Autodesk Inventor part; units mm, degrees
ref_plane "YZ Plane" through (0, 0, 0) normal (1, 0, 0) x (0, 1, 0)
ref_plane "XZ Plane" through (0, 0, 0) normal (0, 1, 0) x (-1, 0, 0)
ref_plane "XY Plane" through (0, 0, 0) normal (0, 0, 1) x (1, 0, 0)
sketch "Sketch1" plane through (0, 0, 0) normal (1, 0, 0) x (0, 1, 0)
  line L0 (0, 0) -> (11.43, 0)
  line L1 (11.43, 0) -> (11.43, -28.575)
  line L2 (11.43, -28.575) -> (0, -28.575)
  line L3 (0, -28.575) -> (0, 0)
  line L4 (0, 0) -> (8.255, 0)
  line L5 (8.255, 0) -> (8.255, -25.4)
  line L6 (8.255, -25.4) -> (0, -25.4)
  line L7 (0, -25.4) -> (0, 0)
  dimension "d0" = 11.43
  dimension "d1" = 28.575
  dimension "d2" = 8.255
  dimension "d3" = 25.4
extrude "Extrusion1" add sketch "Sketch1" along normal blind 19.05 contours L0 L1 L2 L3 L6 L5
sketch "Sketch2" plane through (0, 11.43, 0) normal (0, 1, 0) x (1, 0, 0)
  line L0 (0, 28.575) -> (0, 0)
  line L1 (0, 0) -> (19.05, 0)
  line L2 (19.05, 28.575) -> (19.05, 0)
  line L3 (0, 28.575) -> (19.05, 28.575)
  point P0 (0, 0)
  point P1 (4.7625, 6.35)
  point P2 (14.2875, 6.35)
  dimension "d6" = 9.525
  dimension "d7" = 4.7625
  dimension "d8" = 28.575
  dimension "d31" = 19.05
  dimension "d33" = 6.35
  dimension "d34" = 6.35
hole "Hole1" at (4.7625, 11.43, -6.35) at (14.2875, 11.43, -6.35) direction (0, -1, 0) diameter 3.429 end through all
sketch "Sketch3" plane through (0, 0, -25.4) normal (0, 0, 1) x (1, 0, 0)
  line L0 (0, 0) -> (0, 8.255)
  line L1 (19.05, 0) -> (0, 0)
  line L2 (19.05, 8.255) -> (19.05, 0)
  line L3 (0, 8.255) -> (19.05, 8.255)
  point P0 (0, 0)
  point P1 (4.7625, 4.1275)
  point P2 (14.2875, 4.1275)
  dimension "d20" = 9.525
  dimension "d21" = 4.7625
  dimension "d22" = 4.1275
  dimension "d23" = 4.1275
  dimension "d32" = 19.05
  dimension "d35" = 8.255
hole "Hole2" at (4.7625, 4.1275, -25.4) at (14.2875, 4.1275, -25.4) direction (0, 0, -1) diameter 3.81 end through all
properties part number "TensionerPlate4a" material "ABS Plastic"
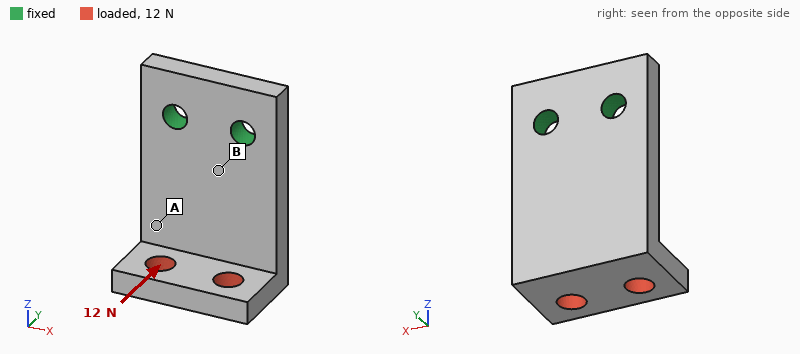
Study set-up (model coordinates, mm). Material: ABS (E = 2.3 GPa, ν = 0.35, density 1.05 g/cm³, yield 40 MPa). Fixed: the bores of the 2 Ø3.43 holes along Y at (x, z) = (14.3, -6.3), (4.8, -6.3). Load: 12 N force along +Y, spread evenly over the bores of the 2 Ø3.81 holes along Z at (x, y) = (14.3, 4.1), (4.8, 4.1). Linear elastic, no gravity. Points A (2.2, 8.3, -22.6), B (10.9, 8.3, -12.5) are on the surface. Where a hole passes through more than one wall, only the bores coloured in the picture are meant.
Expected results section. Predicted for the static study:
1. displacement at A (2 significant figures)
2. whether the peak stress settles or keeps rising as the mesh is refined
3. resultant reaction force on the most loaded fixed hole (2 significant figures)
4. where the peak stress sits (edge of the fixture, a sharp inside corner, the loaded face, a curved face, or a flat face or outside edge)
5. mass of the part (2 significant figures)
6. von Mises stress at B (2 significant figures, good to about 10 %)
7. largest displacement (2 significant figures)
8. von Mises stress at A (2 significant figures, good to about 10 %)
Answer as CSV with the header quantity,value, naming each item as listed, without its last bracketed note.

quantity,value
displacement at A,0.18 mm
whether the peak stress settles or keeps rising as the mesh is refined,keeps rising
resultant reaction force on the most loaded fixed hole,6.0 N
where the peak stress sits,edge of the fixture
mass of the part,2.2 g
von Mises stress at B,4.9 MPa
largest displacement,0.35 mm
von Mises stress at A,1.7 MPa
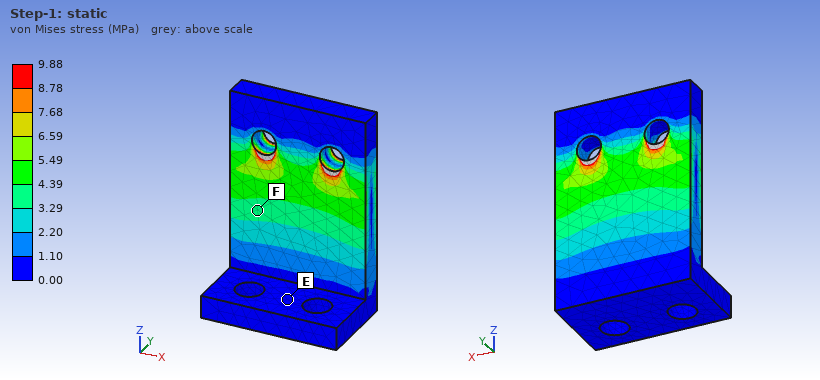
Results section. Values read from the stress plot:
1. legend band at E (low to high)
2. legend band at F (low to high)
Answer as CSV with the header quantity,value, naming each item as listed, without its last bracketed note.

quantity,value
legend band at E,0.00 to 1.10 MPa
legend band at F,3.29 to 4.39 MPa
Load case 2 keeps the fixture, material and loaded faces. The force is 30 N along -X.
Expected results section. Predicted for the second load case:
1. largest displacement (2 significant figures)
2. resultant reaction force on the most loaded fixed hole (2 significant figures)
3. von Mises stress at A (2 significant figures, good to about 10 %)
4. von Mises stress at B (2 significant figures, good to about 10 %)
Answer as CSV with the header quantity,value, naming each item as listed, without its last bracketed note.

quantity,value
largest displacement,0.23 mm
resultant reaction force on the most loaded fixed hole,55 N
von Mises stress at A,4.5 MPa
von Mises stress at B,5.0 MPa
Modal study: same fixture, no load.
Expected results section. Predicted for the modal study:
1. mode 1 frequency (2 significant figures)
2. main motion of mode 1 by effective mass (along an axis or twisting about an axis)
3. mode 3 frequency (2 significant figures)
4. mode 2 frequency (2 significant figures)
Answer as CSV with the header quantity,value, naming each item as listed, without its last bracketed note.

quantity,value
mode 1 frequency,1100 Hz
main motion of mode 1 by effective mass,along Y
mode 3 frequency,4500 Hz
mode 2 frequency,2400 Hz
